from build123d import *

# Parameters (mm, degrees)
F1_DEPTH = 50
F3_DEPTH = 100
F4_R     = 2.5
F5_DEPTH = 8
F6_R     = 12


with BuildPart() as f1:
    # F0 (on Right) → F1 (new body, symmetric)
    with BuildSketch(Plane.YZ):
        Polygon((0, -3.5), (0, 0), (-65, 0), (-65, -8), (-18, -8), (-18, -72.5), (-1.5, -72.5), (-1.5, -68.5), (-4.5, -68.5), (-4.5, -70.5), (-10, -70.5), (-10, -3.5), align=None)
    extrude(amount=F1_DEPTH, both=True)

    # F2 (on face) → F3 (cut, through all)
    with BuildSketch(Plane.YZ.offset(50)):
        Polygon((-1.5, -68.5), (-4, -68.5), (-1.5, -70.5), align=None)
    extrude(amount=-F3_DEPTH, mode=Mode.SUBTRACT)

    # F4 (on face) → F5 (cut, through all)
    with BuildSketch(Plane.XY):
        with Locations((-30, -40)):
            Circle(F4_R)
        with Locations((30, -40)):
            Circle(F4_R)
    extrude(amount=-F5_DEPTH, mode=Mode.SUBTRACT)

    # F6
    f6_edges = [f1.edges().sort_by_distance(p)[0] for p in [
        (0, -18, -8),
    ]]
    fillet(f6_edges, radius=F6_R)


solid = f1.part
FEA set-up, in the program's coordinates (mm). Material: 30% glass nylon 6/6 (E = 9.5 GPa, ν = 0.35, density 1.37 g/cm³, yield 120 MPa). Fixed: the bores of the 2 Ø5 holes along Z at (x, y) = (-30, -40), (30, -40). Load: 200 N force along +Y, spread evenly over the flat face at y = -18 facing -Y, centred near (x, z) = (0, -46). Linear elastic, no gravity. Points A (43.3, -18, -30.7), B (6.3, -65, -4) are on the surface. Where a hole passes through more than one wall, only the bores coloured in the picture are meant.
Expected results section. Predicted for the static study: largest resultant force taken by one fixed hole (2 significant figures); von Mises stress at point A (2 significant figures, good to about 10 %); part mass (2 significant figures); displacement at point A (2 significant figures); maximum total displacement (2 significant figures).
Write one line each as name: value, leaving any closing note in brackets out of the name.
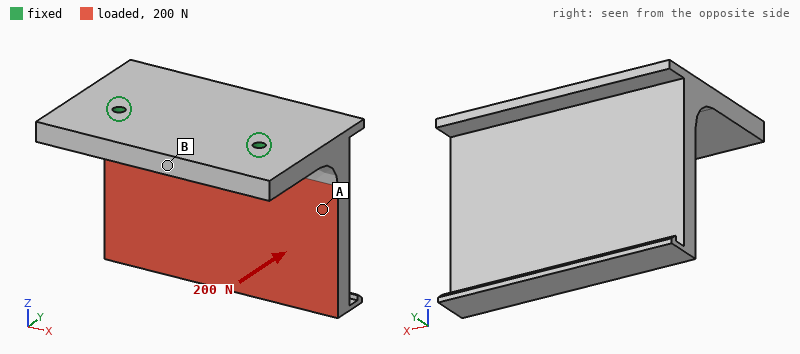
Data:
largest resultant force taken by one fixed hole: 100 N
von Mises stress at point A: 2.8 MPa
part mass: 140 g
displacement at point A: 0.16 mm
maximum total displacement: 0.51 mm
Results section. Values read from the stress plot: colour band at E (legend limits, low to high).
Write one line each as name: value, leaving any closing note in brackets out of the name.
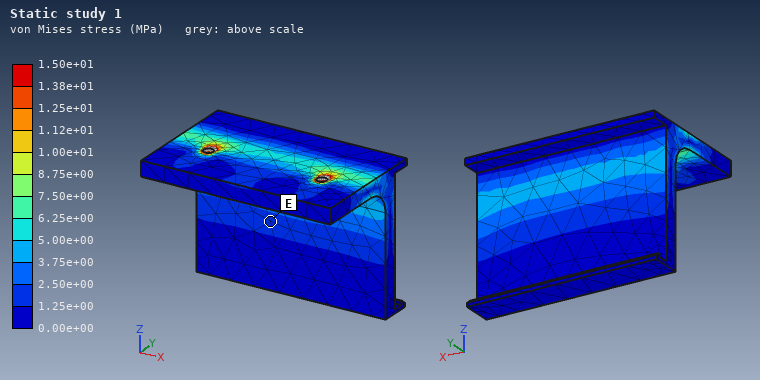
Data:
colour band at E: 1.25e+00 to 2.50e+00 MPa
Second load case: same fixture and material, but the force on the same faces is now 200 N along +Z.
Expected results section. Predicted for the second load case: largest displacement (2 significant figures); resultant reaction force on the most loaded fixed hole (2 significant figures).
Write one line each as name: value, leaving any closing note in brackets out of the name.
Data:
largest displacement: 0.11 mm
resultant reaction force on the most loaded fixed hole: 100 N
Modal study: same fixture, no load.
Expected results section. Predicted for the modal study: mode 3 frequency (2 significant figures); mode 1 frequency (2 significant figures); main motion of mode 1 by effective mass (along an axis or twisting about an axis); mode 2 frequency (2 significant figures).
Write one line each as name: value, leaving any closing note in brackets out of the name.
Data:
mode 3 frequency: 1500 Hz
mode 1 frequency: 460 Hz
main motion of mode 1 by effective mass: along Y
mode 2 frequency: 980 Hz
